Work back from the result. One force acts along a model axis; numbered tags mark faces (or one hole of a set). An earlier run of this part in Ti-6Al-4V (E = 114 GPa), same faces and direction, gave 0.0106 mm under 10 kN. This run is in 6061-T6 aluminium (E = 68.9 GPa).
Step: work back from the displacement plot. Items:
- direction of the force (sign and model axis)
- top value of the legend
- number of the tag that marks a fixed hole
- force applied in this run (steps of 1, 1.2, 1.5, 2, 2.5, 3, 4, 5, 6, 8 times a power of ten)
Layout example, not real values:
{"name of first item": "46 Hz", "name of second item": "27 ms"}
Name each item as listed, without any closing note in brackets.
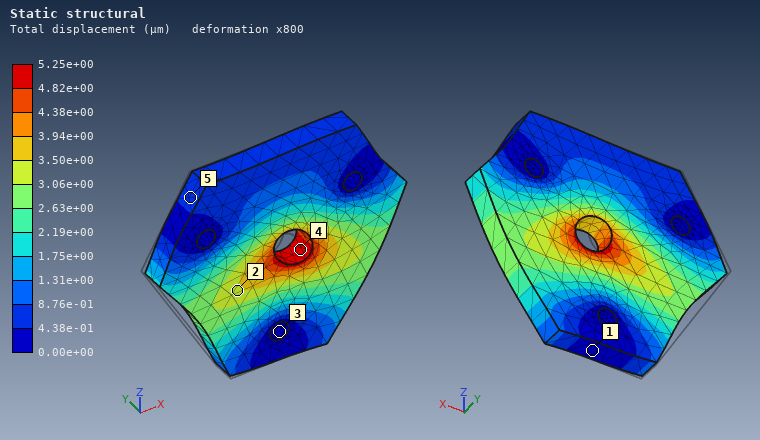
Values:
{"direction of the force": "+X", "top value of the legend": "5.25e+00 µm", "number of the tag that marks a fixed hole": "3", "force applied in this run": "3 kN"}
